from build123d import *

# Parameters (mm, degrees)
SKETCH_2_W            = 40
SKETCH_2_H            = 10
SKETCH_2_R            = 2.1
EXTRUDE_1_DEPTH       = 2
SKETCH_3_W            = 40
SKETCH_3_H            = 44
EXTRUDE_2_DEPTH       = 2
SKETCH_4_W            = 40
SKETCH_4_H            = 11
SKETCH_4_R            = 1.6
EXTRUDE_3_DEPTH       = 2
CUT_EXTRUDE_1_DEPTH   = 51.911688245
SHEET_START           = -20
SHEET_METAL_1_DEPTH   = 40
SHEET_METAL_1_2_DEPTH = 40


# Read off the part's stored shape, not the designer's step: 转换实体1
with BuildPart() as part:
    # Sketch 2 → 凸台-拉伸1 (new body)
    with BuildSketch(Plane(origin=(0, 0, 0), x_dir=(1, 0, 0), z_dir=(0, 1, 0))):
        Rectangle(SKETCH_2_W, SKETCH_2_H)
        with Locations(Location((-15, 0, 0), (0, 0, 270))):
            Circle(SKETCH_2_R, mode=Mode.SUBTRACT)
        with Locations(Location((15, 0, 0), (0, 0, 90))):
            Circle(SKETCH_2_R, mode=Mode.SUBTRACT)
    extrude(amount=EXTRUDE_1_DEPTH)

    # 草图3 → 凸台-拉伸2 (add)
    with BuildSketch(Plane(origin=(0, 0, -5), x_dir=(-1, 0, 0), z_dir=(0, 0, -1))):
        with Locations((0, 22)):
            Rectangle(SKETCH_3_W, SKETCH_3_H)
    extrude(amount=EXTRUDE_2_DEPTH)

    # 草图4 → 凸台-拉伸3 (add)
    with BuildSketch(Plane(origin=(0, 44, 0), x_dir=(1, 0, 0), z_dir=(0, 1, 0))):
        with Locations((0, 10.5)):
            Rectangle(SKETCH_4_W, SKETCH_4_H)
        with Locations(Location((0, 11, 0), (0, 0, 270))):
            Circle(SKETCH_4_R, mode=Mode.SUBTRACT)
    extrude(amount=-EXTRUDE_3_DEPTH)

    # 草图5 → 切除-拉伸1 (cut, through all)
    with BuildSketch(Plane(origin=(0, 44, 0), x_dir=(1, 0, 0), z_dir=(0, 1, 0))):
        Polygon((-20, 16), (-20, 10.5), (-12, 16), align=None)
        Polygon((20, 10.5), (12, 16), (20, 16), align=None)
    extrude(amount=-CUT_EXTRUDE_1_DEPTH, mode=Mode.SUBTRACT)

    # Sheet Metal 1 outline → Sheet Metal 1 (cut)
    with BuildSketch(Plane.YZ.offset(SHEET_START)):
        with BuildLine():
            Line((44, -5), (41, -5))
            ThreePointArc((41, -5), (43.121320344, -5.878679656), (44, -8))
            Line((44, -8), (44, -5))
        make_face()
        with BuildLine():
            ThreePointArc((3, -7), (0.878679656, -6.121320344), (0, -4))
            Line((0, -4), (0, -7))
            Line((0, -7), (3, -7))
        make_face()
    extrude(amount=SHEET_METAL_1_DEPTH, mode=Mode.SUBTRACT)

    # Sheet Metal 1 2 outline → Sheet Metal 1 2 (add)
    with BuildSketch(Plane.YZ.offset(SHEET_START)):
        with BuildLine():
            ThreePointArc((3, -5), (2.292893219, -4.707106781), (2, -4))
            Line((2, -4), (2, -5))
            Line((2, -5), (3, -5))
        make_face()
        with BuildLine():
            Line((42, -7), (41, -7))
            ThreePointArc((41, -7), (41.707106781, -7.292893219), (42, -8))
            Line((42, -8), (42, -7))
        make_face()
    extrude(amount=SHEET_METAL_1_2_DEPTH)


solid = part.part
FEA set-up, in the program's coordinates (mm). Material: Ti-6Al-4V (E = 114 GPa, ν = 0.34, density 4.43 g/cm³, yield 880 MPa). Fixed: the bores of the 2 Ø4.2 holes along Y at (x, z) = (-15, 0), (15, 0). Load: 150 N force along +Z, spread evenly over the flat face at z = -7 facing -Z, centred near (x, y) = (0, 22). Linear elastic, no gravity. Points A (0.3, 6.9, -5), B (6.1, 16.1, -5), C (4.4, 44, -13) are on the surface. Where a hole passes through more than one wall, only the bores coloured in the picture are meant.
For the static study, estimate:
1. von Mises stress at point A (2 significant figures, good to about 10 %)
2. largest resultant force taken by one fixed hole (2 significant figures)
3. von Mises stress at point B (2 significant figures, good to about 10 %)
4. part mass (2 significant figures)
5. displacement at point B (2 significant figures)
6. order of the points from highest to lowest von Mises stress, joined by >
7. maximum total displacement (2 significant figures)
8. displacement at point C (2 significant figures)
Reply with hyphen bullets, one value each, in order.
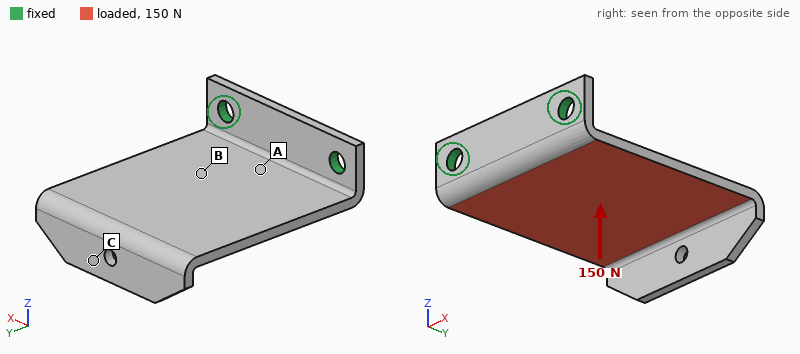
- 77 MPa
- 78 N
- 43 MPa
- 21 g
- 0.16 mm
- A > B > C
- 0.67 mm
- 0.66 mm
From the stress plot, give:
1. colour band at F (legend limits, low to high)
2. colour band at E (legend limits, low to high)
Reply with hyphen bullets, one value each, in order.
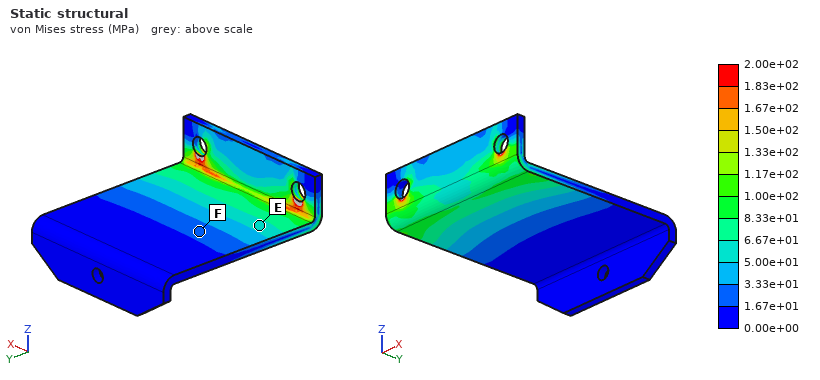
- 1.67e+01 to 3.33e+01 MPa
- 5.00e+01 to 6.67e+01 MPa
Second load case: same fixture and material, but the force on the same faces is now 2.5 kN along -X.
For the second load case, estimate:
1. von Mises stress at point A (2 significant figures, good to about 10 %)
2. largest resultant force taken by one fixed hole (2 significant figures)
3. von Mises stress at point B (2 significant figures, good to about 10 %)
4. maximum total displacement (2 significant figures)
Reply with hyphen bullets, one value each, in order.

- 100 MPa
- 2.2 kN
- 48 MPa
- 0.20 mm
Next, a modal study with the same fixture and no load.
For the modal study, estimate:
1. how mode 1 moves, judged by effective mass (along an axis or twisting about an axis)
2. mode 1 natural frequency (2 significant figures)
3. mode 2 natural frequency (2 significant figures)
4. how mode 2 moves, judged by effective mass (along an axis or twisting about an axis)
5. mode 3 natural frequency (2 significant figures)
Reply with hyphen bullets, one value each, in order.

- along Z
- 600 Hz
- 1800 Hz
- twisting about Y
- 4000 Hz
